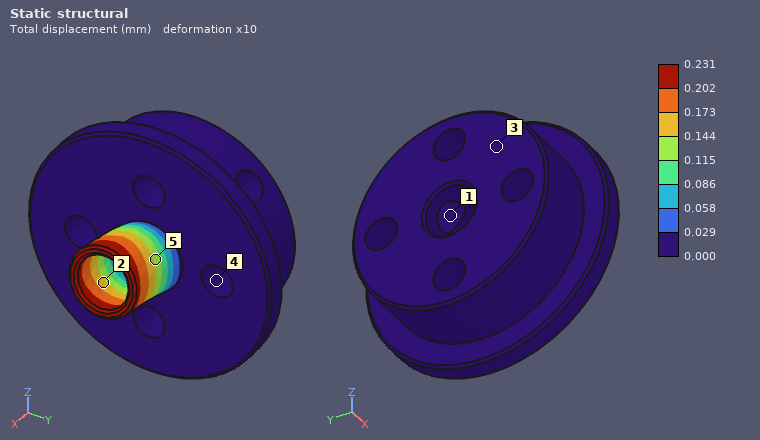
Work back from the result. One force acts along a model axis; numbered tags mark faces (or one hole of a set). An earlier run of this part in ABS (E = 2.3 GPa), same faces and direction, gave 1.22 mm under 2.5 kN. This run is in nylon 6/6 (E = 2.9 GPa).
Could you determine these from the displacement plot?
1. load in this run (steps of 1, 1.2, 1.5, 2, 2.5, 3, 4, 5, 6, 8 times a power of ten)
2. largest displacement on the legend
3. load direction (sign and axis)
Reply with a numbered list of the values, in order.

1. 600 N
2. 0.231 mm
3. +Z
